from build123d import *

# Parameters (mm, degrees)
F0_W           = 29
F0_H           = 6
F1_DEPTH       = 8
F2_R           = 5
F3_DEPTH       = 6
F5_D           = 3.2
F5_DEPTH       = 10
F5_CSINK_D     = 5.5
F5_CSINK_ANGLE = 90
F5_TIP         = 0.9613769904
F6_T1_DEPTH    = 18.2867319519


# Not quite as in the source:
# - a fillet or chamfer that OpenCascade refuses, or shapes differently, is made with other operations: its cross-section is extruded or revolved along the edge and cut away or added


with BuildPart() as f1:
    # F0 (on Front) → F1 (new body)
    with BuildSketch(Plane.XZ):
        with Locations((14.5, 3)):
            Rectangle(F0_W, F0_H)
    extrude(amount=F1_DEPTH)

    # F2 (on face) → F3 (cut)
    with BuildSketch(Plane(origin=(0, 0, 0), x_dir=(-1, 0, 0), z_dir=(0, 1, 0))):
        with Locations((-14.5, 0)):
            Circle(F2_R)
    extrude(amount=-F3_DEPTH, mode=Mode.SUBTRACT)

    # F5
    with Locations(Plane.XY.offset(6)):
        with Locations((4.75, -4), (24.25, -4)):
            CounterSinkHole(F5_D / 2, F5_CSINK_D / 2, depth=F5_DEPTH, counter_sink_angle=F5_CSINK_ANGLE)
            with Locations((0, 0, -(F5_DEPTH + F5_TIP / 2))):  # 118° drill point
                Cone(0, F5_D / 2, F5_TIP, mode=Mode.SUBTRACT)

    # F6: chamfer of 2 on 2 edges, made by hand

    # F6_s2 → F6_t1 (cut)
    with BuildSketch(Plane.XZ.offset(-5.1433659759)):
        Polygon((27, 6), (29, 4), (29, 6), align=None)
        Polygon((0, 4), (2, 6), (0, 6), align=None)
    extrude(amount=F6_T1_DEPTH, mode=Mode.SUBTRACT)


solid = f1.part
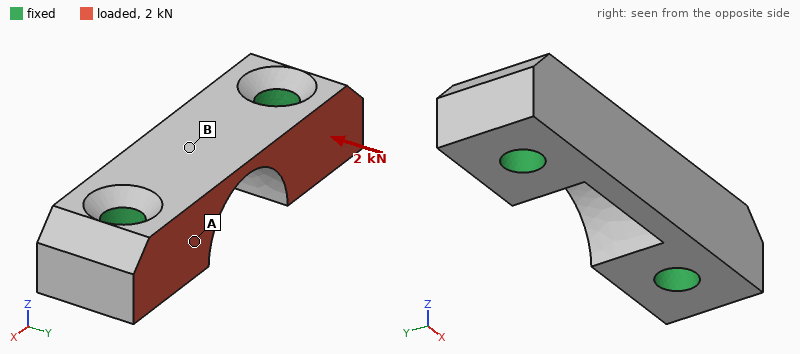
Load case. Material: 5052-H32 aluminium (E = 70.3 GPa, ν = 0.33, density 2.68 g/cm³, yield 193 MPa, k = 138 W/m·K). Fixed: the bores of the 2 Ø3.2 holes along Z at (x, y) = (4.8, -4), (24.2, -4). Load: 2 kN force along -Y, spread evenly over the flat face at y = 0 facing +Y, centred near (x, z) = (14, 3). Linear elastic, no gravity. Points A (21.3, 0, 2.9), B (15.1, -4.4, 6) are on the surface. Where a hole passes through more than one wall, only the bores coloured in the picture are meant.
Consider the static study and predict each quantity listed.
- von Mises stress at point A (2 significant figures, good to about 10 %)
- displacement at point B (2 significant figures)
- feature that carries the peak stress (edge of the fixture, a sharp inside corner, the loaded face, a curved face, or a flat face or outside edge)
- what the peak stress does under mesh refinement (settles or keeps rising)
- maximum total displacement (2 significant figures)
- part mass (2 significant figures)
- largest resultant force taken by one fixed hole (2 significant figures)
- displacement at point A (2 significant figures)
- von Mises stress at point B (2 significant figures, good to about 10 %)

22 MPa
4.5 µm
edge of the fixture
keeps rising
6.0 µm
2.7 g
1.0 kN
2.4 µm
10 MPa
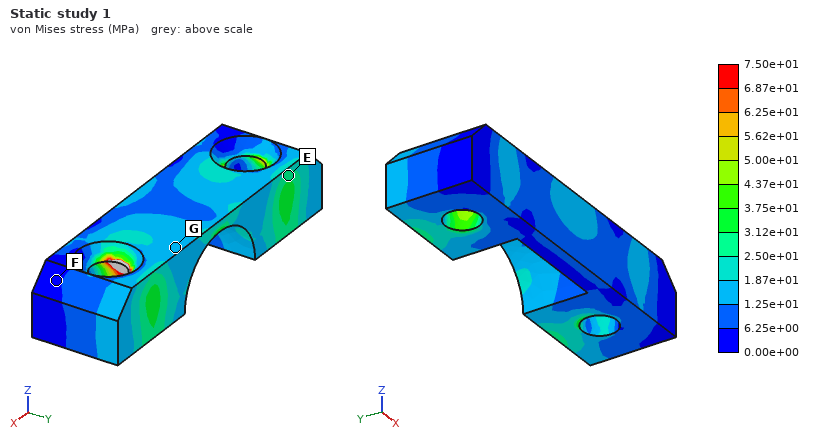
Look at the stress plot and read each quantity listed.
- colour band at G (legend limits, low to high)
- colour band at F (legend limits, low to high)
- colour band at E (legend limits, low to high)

1.25e+01 to 1.87e+01 MPa
0.00e+00 to 6.25e+00 MPa
2.50e+01 to 3.12e+01 MPa
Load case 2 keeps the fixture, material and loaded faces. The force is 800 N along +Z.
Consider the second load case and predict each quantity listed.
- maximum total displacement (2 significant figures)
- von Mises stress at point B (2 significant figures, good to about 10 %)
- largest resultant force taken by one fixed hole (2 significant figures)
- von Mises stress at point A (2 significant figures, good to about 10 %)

7.0 µm
8.3 MPa
400 N
19 MPa
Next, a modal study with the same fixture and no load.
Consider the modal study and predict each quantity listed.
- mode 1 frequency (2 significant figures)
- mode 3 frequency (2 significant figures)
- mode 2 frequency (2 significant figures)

64 kHz
81 kHz
67 kHz
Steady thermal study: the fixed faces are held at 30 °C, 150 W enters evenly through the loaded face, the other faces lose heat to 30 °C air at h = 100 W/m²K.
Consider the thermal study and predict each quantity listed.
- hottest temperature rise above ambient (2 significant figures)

52 K
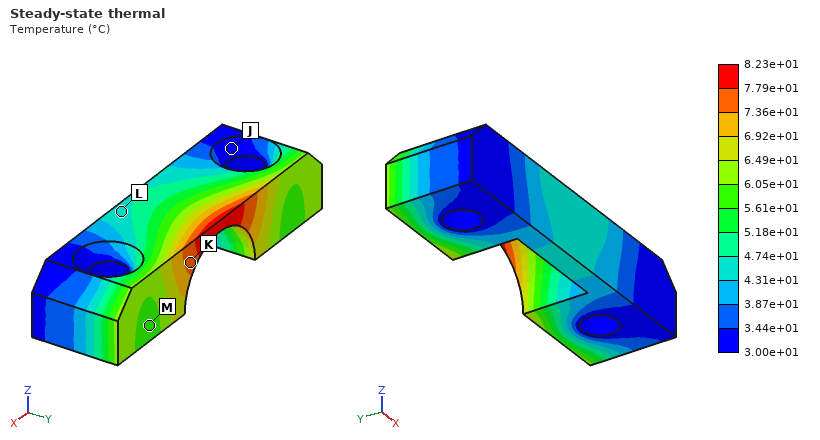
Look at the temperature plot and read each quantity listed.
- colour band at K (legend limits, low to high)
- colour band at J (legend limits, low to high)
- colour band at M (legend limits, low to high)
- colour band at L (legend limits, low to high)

7.36e+01 to 7.79e+01 °C
3.00e+01 to 3.44e+01 °C
5.61e+01 to 6.05e+01 °C
4.31e+01 to 4.74e+01 °C
